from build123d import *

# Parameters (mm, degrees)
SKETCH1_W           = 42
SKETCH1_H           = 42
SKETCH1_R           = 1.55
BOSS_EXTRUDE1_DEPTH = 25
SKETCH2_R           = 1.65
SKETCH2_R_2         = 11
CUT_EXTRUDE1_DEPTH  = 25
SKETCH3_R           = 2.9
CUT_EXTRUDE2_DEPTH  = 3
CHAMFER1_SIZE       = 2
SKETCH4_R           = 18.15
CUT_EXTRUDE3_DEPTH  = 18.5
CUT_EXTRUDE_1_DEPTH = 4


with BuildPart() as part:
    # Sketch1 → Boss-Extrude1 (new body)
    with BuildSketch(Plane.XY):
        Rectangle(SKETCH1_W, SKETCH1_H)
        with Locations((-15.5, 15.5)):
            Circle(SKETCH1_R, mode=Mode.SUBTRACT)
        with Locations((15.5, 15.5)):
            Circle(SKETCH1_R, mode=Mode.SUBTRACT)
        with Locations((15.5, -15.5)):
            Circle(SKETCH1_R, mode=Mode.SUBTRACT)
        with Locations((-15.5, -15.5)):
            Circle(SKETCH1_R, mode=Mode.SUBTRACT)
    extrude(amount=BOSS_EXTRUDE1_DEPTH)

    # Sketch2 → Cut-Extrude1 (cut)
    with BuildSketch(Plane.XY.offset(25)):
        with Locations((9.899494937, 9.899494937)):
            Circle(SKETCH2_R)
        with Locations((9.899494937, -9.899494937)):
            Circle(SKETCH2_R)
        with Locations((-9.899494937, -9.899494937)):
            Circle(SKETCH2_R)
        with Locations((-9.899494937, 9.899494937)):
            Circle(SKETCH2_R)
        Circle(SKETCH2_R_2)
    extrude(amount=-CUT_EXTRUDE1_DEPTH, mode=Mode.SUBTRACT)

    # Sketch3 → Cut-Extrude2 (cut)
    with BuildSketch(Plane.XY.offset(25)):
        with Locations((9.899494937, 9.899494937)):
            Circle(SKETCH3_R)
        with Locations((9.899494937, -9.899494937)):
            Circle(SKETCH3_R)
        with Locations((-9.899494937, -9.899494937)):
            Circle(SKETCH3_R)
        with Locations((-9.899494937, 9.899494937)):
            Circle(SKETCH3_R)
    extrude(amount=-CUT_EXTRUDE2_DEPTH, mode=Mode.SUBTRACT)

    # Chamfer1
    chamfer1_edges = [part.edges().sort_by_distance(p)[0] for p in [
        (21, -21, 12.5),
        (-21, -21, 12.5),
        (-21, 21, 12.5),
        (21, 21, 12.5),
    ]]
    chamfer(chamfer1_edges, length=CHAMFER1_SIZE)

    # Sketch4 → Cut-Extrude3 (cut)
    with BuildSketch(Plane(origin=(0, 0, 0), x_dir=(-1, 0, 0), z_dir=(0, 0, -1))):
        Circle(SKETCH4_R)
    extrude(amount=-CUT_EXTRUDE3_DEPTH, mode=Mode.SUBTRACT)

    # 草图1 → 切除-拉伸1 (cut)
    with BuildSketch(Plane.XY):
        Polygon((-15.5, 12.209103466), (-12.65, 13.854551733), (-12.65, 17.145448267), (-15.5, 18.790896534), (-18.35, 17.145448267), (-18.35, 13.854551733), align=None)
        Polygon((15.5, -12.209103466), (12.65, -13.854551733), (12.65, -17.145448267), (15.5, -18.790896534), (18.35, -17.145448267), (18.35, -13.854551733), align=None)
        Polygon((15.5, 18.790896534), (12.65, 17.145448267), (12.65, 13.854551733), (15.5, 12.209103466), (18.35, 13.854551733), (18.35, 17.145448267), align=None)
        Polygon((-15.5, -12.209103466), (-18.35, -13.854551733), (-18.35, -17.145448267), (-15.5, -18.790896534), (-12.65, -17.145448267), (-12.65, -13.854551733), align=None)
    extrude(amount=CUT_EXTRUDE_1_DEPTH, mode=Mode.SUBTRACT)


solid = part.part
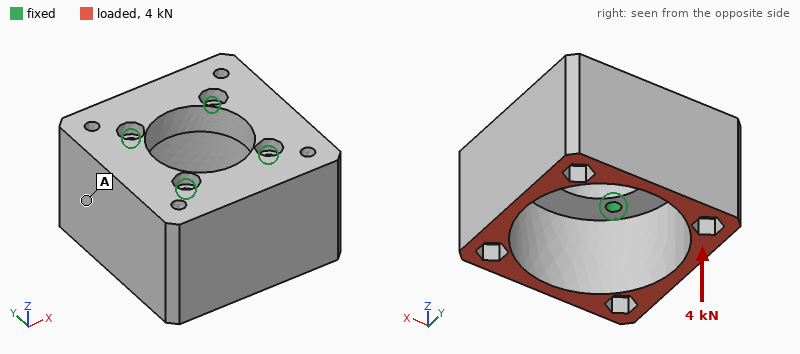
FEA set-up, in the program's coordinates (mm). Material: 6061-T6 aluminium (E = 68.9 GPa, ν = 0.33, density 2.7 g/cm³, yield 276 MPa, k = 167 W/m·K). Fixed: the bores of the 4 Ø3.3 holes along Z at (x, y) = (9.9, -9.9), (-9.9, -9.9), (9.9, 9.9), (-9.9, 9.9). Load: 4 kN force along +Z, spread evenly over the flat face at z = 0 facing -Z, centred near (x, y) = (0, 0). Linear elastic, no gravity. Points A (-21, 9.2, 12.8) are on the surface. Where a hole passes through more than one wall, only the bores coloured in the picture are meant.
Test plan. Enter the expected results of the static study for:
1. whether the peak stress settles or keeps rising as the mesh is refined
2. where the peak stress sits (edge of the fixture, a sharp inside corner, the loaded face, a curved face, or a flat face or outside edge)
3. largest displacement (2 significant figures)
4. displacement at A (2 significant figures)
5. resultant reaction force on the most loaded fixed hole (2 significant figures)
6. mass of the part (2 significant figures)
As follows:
keeps rising
edge of the fixture
10 µm
8.6 µm
1.0 kN
56 g
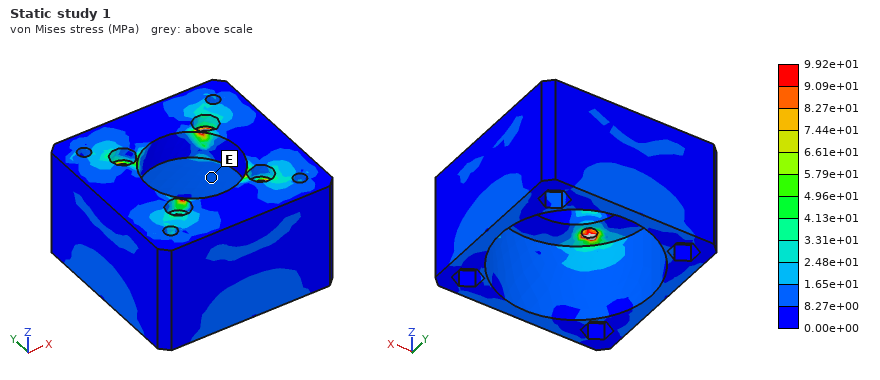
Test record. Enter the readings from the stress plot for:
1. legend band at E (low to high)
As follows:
8.27e+00 to 1.65e+01 MPa
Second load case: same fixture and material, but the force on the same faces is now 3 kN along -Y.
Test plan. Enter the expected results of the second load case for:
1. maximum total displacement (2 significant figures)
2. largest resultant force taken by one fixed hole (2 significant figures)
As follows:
50 µm
1.5 kN
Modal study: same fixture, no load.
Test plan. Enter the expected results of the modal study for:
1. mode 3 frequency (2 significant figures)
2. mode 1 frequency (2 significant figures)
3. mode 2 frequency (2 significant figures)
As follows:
9600 Hz
9500 Hz
9500 Hz
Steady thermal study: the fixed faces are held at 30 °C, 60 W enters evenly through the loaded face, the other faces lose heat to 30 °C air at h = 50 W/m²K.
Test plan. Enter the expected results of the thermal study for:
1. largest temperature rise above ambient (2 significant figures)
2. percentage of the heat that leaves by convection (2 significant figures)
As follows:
17 K
7.8 %
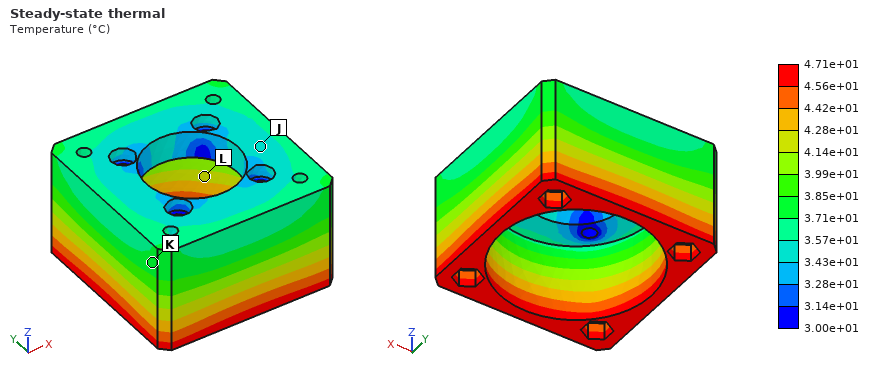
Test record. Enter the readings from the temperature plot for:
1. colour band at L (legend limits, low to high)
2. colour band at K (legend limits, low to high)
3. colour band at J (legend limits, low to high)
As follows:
4.14e+01 to 4.28e+01 °C
3.71e+01 to 3.85e+01 °C
3.43e+01 to 3.57e+01 °C
